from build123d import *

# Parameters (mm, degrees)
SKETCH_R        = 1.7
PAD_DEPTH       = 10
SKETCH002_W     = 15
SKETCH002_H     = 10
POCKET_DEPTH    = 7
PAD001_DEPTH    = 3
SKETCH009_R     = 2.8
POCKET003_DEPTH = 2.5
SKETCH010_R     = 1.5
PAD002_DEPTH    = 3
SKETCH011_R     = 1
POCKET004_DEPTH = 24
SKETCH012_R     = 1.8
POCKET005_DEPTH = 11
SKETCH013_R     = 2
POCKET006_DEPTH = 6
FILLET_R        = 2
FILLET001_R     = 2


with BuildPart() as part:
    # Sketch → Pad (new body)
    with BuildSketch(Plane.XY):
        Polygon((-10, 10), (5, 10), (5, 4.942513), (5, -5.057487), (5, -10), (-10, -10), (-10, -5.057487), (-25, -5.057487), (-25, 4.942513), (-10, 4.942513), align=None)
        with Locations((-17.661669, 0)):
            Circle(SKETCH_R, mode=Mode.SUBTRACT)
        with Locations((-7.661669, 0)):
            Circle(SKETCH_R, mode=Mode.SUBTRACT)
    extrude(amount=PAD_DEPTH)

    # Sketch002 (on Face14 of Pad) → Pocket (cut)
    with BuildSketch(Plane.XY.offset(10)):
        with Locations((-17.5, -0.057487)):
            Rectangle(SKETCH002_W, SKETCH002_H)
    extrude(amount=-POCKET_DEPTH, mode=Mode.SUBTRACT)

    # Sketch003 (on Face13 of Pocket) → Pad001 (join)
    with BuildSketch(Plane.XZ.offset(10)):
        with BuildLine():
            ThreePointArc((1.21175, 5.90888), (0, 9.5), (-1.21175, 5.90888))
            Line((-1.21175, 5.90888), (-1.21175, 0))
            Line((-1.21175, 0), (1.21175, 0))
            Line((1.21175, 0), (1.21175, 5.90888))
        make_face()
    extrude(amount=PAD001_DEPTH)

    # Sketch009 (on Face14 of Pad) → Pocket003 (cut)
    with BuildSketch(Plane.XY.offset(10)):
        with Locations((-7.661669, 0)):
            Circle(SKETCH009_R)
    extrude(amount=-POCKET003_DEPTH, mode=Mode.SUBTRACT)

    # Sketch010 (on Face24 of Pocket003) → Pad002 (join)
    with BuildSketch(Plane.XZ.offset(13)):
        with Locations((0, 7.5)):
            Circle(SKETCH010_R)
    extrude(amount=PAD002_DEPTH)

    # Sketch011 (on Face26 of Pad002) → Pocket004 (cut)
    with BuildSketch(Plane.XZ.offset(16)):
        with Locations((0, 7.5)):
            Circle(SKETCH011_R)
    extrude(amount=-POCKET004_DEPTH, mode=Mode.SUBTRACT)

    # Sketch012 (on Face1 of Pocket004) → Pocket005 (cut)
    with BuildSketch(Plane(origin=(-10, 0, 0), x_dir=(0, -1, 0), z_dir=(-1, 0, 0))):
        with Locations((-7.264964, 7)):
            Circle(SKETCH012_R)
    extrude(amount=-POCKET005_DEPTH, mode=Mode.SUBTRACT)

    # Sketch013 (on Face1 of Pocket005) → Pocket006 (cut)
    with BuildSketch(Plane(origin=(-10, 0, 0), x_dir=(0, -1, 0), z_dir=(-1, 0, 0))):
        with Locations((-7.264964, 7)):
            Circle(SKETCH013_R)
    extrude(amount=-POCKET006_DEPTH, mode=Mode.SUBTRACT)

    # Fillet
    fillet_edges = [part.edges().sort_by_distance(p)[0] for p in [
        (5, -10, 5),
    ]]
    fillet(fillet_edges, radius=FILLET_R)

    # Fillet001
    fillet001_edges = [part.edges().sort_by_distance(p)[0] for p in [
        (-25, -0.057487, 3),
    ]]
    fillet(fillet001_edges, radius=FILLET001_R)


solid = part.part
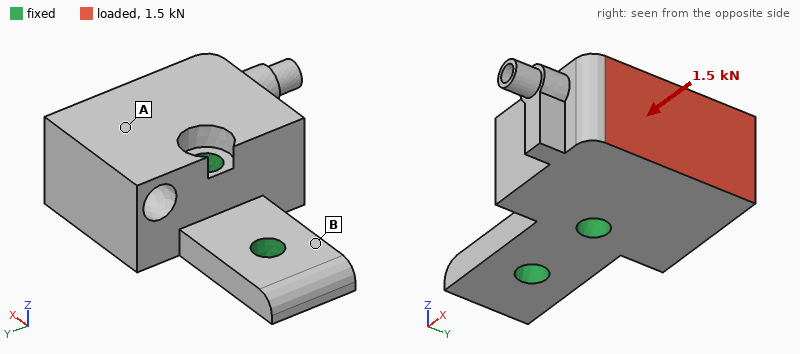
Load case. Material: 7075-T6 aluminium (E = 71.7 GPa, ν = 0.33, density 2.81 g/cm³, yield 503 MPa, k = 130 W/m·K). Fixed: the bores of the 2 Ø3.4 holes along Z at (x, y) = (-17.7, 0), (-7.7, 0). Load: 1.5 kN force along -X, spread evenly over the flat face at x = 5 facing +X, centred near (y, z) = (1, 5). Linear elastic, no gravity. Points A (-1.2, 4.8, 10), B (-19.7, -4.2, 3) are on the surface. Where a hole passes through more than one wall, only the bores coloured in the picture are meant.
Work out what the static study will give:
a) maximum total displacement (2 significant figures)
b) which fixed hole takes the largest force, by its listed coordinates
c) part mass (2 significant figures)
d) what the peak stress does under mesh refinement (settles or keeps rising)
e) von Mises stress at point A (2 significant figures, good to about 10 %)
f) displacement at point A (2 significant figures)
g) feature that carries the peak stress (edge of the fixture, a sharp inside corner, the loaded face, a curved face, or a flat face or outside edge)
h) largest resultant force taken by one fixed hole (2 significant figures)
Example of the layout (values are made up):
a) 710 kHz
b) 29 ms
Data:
a) 8.2 µm
b) (-7.7, 0)
c) 8.9 g
d) keeps rising
e) 12 MPa
f) 5.0 µm
g) edge of the fixture
h) 1.4 kN
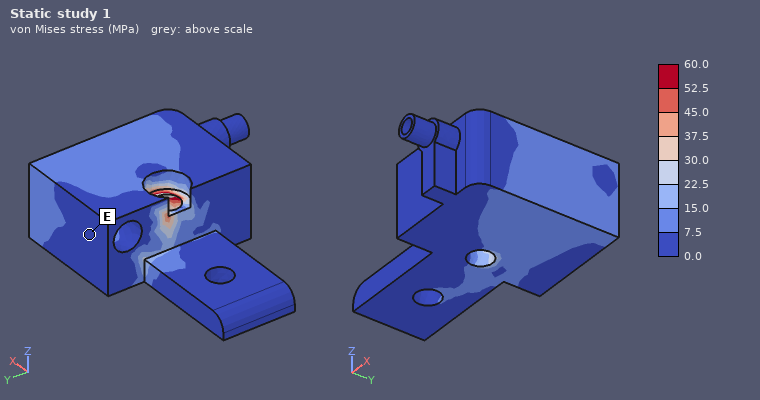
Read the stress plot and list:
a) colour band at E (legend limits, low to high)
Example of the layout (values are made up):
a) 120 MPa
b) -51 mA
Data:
a) 0.0 to 7.5 MPa
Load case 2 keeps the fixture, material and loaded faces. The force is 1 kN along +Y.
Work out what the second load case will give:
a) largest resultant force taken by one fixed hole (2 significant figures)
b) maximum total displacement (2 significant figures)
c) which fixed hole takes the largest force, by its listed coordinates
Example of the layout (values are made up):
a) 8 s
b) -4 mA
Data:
a) 1.4 kN
b) 30 µm
c) (-7.7, 0)
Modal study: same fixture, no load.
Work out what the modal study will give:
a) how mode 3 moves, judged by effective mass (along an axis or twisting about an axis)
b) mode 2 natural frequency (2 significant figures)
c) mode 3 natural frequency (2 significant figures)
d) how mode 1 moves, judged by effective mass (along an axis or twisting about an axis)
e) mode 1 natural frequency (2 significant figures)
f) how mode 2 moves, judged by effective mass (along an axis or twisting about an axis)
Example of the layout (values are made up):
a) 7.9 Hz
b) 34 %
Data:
a) twisting about X
b) 21 kHz
c) 26 kHz
d) along Y
e) 18 kHz
f) along Z
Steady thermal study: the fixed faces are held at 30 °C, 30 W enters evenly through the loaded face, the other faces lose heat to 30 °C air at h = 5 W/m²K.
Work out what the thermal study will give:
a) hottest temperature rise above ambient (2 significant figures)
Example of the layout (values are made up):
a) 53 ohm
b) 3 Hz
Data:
a) 22 K
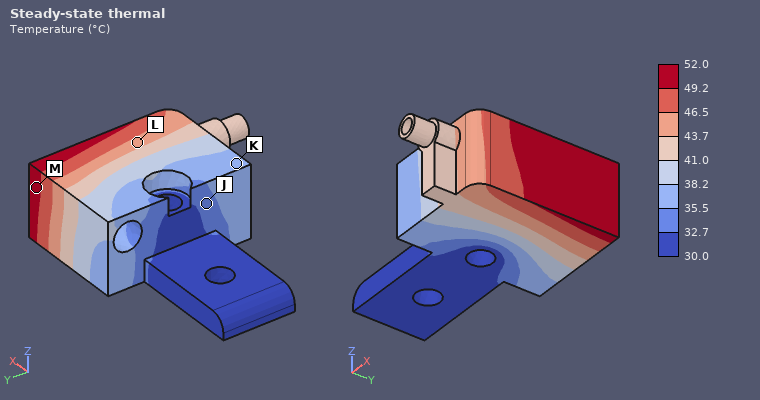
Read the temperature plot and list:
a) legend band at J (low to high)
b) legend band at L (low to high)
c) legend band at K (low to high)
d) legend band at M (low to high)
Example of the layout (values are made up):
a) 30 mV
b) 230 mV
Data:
a) 32.7 to 35.5 °C
b) 43.7 to 46.5 °C
c) 35.5 to 38.2 °C
d) 49.2 to 52.0 °C
